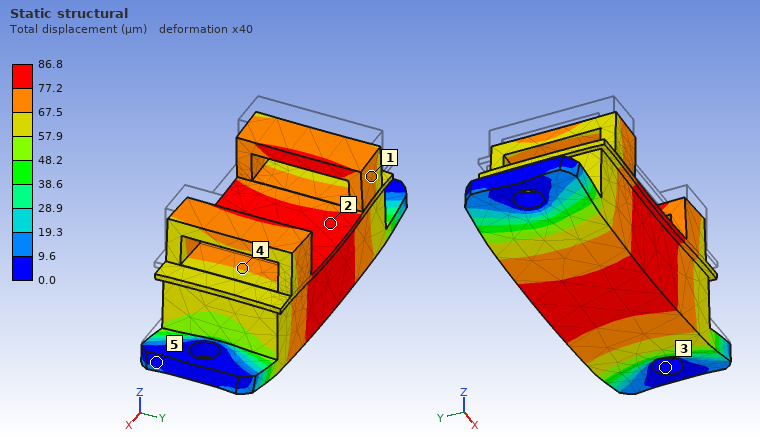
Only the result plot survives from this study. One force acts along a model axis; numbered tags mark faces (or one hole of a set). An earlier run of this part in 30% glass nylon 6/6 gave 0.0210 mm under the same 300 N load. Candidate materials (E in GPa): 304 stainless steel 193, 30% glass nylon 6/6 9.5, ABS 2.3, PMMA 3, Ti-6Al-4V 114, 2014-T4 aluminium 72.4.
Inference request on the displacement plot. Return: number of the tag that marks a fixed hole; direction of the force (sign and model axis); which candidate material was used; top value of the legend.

3
-Z
ABS
86.8 µm
